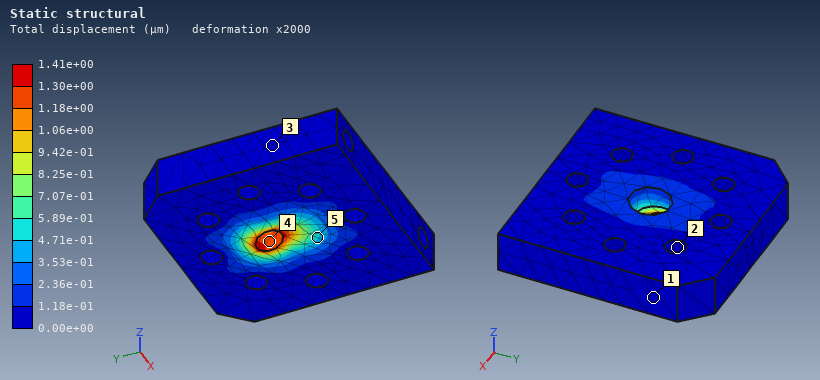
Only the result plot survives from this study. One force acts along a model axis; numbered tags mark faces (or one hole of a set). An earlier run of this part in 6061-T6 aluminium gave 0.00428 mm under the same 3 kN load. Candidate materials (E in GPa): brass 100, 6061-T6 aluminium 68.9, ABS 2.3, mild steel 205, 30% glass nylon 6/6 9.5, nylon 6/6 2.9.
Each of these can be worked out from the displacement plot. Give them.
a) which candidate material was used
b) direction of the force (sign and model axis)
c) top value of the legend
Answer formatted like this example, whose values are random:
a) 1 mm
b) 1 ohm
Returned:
a) mild steel
b) +Y
c) 1.41e+00 µm
